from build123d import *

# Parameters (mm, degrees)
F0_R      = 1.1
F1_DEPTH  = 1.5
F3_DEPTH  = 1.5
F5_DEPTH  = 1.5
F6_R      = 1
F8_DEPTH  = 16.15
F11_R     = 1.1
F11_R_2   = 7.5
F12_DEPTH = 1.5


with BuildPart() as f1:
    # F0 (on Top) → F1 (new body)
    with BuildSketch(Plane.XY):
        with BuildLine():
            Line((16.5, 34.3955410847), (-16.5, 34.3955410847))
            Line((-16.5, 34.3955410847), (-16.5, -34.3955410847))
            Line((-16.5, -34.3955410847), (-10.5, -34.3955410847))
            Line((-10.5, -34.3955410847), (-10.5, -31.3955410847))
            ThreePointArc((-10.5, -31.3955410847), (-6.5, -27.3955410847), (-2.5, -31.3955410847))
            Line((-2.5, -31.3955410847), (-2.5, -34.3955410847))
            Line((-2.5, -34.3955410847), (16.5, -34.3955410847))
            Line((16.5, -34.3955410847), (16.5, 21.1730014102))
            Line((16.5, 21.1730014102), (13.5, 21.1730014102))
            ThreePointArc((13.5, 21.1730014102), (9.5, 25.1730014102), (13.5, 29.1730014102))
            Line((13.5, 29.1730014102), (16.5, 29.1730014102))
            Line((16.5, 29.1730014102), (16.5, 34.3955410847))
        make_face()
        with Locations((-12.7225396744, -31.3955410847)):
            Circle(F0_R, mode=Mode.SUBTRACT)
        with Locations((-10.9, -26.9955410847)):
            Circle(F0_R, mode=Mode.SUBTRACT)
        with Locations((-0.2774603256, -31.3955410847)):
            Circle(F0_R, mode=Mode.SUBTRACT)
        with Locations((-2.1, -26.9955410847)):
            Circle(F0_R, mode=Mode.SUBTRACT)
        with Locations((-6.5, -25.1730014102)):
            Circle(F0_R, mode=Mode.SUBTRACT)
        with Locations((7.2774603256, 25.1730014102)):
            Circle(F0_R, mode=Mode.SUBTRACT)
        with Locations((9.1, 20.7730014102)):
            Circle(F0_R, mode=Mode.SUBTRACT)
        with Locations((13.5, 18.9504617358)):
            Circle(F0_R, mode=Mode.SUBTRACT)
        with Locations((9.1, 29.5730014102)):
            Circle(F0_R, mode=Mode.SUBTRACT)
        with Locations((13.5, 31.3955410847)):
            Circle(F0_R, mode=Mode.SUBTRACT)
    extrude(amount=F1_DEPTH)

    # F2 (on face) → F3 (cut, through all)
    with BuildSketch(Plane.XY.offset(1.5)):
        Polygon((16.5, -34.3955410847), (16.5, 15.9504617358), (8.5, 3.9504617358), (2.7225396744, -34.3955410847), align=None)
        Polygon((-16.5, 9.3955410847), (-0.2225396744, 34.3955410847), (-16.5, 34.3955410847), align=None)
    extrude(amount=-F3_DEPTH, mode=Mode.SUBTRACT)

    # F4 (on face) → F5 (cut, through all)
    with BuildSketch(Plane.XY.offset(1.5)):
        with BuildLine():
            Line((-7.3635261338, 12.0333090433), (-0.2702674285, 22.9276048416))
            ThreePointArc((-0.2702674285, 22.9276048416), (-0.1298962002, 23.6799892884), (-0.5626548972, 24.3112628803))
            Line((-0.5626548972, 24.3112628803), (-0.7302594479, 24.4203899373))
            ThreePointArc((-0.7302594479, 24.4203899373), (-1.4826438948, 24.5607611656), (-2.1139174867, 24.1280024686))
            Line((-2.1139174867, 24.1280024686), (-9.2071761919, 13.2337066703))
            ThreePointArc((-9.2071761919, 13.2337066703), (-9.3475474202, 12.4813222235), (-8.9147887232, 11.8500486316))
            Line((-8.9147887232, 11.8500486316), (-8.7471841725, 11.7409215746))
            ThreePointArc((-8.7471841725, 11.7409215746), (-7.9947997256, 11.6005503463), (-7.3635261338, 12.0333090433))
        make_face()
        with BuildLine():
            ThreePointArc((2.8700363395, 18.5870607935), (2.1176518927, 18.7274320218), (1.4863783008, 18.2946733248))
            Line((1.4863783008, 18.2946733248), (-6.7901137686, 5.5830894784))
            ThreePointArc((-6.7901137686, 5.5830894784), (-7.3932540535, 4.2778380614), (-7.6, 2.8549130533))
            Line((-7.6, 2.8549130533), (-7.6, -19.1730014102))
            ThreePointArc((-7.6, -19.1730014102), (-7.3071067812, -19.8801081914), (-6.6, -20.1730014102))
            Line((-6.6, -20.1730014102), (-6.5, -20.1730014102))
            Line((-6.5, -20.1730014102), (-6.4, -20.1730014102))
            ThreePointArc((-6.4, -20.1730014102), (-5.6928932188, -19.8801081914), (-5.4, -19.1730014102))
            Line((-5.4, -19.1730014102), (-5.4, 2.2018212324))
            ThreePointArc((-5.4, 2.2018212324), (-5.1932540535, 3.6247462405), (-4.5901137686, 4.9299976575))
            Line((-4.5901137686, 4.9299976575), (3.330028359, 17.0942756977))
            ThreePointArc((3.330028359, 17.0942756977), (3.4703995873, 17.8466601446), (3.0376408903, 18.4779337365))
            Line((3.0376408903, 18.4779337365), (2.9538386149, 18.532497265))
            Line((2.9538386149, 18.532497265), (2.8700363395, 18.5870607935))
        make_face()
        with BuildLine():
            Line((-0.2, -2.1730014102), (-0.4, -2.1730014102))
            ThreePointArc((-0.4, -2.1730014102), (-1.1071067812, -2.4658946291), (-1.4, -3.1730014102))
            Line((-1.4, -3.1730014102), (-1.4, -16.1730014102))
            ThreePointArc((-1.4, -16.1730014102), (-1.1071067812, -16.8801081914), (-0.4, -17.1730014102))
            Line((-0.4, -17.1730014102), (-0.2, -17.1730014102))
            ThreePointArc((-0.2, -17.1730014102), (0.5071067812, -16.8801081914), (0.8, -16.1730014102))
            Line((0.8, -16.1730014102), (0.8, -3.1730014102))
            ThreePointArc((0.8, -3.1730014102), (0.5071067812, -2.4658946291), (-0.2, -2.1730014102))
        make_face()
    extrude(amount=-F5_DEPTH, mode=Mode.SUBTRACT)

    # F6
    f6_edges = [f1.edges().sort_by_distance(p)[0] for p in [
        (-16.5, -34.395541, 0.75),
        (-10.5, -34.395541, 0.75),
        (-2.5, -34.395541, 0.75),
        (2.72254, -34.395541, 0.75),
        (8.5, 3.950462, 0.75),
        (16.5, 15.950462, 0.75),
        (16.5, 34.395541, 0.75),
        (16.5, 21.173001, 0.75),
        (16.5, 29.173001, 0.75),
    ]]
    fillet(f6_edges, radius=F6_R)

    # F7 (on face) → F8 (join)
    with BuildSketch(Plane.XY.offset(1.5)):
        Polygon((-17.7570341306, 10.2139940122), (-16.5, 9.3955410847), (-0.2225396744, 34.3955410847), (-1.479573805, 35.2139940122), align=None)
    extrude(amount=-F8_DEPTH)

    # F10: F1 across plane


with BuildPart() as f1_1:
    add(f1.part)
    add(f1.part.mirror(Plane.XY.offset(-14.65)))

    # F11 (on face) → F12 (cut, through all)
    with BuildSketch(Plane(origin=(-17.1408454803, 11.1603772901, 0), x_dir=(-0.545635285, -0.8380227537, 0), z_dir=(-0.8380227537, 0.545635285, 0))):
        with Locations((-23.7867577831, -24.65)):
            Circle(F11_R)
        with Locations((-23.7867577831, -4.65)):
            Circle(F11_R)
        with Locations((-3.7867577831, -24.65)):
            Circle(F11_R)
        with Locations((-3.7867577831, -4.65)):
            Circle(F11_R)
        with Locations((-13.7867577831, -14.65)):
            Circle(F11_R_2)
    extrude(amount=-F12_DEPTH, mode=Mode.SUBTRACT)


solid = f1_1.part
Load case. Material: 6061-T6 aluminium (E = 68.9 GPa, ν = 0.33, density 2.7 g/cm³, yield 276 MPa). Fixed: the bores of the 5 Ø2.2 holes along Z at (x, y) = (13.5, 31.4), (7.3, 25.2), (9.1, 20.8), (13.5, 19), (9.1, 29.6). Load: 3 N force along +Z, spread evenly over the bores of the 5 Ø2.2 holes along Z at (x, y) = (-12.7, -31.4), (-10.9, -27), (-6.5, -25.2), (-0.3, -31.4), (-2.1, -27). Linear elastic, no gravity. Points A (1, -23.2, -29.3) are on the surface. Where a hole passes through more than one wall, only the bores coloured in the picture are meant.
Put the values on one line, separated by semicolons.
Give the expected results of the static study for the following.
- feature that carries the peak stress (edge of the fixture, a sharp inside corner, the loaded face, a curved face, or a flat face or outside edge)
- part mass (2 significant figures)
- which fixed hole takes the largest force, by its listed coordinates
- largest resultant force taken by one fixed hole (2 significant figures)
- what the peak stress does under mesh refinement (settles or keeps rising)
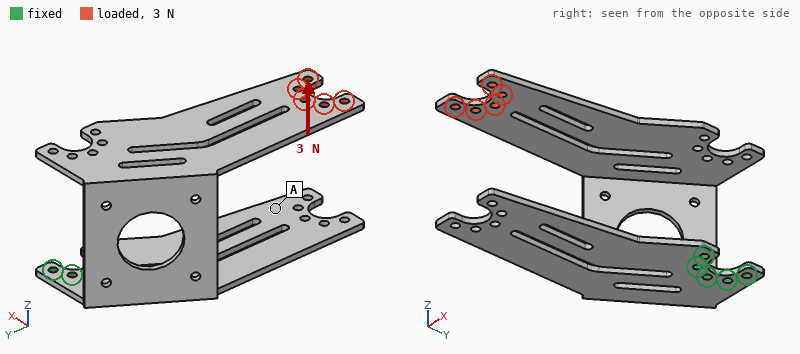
a sharp inside corner; 14 g; (9.1, 29.6); 15 N; keeps rising
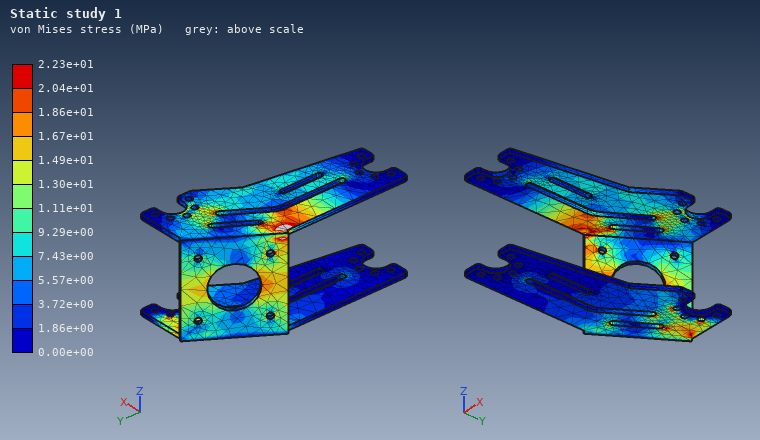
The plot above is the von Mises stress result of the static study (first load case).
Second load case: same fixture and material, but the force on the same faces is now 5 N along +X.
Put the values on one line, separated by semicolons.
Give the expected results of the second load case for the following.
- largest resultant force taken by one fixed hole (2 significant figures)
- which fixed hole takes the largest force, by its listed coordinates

19 N; (7.3, 25.2)
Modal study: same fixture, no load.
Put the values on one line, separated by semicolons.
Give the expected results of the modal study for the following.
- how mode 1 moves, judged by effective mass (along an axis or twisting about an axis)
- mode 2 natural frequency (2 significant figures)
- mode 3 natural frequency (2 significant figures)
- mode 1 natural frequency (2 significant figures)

along X; 270 Hz; 490 Hz; 210 Hz
